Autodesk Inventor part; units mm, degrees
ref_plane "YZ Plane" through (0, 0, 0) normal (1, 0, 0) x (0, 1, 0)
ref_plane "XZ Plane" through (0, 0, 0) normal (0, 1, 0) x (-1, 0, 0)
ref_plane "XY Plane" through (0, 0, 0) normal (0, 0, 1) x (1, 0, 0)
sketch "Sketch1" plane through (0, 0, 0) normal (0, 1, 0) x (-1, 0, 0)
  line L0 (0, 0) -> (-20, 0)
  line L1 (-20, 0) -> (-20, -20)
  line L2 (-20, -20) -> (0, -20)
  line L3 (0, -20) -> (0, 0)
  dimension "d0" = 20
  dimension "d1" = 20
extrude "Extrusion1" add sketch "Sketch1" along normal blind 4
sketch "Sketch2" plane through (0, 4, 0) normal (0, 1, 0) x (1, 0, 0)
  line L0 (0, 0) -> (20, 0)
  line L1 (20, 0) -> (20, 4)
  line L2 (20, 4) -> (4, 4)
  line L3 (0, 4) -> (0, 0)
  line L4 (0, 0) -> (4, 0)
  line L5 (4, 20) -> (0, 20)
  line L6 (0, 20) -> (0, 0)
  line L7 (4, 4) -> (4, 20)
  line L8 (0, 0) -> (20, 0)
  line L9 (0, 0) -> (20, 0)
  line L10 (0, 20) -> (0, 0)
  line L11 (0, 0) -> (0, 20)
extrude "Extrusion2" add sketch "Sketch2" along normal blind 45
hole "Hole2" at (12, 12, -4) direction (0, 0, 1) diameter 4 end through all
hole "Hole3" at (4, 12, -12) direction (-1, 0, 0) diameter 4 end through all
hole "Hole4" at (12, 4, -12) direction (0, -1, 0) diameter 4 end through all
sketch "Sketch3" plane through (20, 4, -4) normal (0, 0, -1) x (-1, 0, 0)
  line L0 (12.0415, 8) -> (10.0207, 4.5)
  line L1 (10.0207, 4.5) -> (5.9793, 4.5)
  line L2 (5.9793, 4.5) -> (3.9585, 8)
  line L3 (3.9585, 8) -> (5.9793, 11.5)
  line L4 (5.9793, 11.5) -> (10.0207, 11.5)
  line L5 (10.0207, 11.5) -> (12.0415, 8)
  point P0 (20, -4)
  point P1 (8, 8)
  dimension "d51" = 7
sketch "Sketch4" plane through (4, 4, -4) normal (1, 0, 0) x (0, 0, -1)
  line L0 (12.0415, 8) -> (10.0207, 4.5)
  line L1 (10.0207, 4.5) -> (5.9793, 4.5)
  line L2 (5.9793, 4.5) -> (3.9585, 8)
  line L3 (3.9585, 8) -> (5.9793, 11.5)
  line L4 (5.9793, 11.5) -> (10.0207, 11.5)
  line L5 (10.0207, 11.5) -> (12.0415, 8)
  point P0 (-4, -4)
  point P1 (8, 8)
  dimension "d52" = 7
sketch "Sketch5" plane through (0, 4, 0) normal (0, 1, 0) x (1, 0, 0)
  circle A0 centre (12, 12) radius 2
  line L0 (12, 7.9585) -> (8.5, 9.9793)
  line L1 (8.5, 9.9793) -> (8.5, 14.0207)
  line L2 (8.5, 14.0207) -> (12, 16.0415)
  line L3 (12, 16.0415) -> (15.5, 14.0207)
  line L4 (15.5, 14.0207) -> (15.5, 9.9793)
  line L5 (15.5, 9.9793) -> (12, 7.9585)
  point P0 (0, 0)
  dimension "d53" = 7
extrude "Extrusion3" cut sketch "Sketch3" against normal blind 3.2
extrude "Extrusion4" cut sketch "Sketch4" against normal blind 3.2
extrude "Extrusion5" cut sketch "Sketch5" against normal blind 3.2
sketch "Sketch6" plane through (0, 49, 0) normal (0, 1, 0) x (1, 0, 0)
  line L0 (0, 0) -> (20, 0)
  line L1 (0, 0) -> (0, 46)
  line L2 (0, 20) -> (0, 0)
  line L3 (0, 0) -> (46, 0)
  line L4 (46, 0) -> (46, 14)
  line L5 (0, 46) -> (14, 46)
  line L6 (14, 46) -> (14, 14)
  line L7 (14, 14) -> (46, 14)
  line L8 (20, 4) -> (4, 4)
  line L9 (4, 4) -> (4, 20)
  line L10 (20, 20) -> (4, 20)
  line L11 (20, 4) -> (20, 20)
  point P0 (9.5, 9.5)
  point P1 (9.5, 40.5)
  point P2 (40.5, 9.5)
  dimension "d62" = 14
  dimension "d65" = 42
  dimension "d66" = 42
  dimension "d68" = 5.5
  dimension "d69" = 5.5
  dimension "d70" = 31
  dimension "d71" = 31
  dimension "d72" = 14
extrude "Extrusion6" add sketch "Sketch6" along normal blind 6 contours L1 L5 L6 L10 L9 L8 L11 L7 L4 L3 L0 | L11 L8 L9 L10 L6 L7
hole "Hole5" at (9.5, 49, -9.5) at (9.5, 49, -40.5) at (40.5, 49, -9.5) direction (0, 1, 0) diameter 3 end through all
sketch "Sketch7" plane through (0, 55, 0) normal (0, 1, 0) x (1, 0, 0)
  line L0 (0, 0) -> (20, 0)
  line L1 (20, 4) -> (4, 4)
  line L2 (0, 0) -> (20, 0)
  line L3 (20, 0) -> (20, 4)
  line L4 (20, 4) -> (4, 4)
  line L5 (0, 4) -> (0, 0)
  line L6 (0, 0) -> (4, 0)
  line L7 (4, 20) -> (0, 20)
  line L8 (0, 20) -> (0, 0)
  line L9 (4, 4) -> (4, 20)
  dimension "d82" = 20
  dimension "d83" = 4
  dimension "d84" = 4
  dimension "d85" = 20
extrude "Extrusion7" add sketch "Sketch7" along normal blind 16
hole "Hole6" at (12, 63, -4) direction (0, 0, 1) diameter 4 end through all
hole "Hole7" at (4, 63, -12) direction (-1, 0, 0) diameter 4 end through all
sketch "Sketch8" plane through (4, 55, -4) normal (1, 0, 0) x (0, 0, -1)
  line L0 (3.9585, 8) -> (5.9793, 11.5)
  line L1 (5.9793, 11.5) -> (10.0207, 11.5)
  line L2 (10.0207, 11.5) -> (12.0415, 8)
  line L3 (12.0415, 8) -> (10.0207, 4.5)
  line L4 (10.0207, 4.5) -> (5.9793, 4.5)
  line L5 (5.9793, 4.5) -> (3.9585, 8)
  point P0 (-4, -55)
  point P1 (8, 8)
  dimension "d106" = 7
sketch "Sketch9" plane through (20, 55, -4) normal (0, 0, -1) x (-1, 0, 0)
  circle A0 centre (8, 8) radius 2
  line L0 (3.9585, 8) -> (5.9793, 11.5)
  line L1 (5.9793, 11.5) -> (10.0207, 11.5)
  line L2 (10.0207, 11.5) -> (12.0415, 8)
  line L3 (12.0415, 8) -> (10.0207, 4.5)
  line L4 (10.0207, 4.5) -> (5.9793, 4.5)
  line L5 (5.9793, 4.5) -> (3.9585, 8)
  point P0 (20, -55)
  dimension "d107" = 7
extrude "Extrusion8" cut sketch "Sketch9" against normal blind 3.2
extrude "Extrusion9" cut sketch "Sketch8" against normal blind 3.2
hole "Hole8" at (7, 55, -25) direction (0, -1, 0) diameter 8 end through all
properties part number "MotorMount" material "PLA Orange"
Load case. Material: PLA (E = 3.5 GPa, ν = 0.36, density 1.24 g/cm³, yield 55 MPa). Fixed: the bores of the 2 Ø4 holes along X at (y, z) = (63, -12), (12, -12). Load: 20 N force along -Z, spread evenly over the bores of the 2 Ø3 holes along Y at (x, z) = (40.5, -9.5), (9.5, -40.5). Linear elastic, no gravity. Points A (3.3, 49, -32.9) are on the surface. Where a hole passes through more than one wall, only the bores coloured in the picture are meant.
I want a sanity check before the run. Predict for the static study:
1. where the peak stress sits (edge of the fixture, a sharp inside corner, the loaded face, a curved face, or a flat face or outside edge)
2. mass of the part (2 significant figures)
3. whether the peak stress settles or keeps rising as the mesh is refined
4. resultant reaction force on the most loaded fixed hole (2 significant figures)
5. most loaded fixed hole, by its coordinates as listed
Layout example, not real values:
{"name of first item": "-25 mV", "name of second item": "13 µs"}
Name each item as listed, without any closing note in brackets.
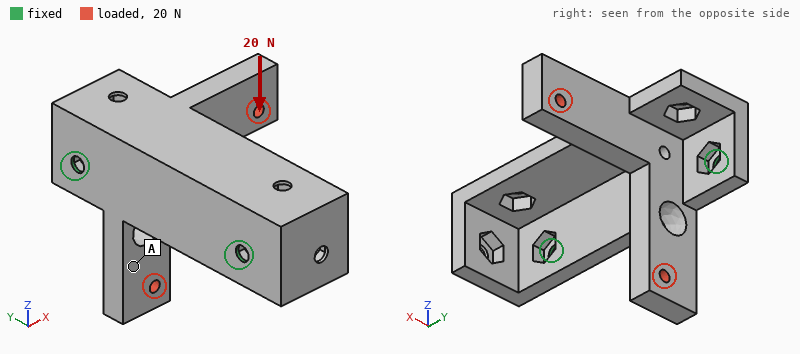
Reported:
{"where the peak stress sits": "edge of the fixture", "mass of the part": "20 g", "whether the peak stress settles or keeps rising as the mesh is refined": "keeps rising", "resultant reaction force on the most loaded fixed hole": "18 N", "most loaded fixed hole, by its coordinates as listed": "(63, -12)"}
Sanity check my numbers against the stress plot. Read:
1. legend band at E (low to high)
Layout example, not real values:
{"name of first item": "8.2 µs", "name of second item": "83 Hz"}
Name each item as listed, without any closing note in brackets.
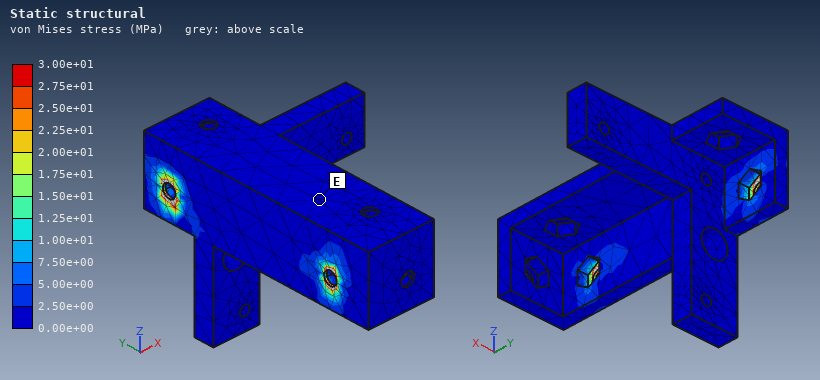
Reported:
{"legend band at E": "0.00e+00 to 2.50e+00 MPa"}
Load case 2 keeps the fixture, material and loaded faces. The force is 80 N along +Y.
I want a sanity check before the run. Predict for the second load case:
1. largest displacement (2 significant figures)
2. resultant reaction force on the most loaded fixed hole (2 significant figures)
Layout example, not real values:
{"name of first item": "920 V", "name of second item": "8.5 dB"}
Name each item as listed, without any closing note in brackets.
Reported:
{"largest displacement": "0.75 mm", "resultant reaction force on the most loaded fixed hole": "62 N"}
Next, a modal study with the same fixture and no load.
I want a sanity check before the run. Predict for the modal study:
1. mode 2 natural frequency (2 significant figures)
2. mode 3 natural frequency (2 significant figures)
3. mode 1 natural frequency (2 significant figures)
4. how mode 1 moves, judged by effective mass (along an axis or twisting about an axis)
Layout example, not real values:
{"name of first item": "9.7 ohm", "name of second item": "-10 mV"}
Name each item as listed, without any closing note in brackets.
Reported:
{"mode 2 natural frequency": "990 Hz", "mode 3 natural frequency": "1300 Hz", "mode 1 natural frequency": "290 Hz", "how mode 1 moves, judged by effective mass": "along Z"}
